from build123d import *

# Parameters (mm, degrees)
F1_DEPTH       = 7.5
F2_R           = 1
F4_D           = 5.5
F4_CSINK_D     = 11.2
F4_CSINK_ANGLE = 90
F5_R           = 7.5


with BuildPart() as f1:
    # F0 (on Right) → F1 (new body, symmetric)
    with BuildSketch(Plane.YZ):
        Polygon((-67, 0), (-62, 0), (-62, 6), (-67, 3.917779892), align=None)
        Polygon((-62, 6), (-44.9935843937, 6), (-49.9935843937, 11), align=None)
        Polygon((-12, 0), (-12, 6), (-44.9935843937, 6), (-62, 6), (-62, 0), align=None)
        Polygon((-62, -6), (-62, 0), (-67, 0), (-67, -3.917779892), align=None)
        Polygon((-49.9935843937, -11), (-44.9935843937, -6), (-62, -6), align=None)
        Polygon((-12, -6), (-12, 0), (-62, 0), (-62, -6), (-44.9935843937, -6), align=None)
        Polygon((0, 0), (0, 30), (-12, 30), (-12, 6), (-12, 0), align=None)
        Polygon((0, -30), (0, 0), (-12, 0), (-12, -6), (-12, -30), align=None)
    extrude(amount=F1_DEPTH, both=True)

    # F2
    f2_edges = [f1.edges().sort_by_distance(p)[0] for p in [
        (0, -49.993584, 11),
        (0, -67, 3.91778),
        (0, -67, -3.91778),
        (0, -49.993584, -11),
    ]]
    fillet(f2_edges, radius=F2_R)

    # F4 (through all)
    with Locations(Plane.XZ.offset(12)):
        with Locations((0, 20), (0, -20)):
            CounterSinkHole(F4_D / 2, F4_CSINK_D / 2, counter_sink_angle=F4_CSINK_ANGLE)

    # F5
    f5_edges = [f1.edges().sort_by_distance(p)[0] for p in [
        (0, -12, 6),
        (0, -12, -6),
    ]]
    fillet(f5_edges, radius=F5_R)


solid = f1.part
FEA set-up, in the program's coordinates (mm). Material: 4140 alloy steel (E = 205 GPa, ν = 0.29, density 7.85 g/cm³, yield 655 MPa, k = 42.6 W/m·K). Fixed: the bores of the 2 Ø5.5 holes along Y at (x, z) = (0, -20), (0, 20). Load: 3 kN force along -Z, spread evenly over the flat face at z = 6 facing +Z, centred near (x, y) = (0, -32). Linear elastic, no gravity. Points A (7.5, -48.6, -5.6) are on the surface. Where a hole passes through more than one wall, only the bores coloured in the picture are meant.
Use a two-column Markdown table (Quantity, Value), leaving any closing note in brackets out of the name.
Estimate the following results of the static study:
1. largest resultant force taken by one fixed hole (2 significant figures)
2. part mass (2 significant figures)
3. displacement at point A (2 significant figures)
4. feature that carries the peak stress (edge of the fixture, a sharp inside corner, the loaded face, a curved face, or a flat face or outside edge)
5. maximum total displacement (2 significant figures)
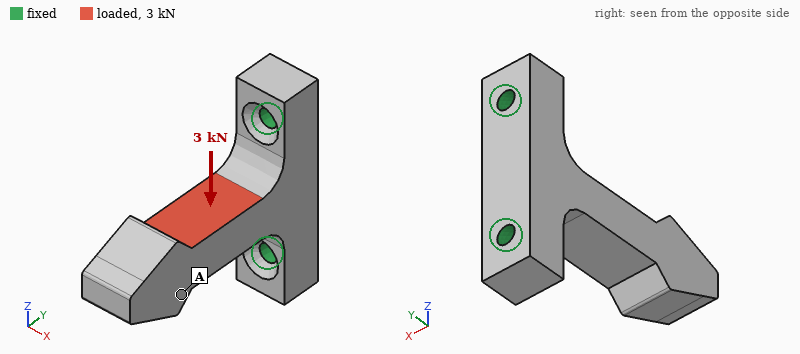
| Quantity | Value |
|---|---|
| largest resultant force taken by one fixed hole | 2.8 kN |
| part mass | 170 g |
| displacement at point A | 53 µm |
| feature that carries the peak stress | a curved face |
| maximum total displacement | 83 µm |
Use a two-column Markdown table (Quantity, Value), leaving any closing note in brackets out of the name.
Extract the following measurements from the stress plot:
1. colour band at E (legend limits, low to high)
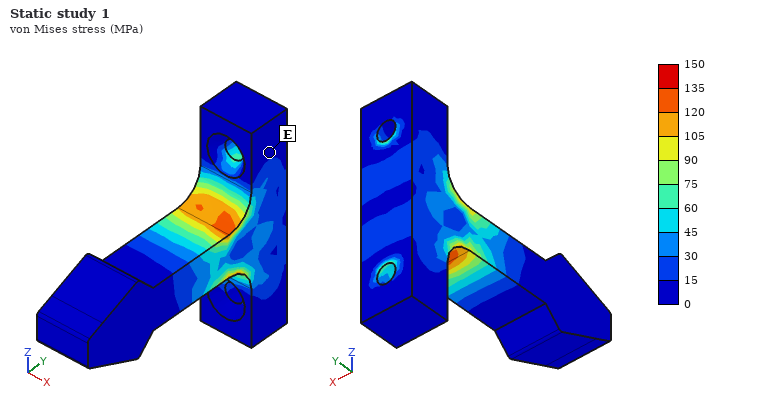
| Quantity | Value |
|---|---|
| colour band at E | 0 to 15 MPa |
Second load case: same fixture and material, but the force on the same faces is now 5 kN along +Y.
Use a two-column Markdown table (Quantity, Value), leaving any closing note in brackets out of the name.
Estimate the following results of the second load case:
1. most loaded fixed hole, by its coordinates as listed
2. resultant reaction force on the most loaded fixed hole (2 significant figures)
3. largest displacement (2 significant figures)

| Quantity | Value |
|---|---|
| most loaded fixed hole, by its coordinates as listed | (0, 20) |
| resultant reaction force on the most loaded fixed hole | 3.6 kN |
| largest displacement | 62 µm |
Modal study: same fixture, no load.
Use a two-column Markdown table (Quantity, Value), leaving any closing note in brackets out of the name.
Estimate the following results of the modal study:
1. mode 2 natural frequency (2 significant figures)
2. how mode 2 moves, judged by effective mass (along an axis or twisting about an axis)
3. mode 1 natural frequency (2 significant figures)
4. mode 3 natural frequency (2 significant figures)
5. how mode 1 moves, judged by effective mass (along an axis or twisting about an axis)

| Quantity | Value |
|---|---|
| mode 2 natural frequency | 2900 Hz |
| how mode 2 moves, judged by effective mass | along Z |
| mode 1 natural frequency | 2300 Hz |
| mode 3 natural frequency | 11 kHz |
| how mode 1 moves, judged by effective mass | along X |
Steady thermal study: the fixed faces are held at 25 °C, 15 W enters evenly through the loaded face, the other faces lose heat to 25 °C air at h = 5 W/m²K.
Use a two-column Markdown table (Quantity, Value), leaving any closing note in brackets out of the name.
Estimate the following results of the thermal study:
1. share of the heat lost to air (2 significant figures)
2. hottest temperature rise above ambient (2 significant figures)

| Quantity | Value |
|---|---|
| share of the heat lost to air | 4.9 % |
| hottest temperature rise above ambient | 55 K |
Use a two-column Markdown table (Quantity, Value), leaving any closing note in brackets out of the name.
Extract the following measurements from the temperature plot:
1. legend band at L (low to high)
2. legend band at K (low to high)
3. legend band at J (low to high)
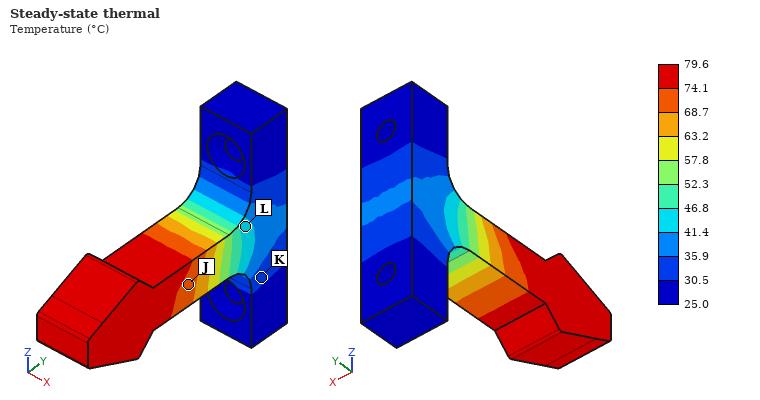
| Quantity | Value |
|---|---|
| legend band at L | 41.4 to 46.8 °C |
| legend band at K | 30.5 to 35.9 °C |
| legend band at J | 68.7 to 74.1 °C |
